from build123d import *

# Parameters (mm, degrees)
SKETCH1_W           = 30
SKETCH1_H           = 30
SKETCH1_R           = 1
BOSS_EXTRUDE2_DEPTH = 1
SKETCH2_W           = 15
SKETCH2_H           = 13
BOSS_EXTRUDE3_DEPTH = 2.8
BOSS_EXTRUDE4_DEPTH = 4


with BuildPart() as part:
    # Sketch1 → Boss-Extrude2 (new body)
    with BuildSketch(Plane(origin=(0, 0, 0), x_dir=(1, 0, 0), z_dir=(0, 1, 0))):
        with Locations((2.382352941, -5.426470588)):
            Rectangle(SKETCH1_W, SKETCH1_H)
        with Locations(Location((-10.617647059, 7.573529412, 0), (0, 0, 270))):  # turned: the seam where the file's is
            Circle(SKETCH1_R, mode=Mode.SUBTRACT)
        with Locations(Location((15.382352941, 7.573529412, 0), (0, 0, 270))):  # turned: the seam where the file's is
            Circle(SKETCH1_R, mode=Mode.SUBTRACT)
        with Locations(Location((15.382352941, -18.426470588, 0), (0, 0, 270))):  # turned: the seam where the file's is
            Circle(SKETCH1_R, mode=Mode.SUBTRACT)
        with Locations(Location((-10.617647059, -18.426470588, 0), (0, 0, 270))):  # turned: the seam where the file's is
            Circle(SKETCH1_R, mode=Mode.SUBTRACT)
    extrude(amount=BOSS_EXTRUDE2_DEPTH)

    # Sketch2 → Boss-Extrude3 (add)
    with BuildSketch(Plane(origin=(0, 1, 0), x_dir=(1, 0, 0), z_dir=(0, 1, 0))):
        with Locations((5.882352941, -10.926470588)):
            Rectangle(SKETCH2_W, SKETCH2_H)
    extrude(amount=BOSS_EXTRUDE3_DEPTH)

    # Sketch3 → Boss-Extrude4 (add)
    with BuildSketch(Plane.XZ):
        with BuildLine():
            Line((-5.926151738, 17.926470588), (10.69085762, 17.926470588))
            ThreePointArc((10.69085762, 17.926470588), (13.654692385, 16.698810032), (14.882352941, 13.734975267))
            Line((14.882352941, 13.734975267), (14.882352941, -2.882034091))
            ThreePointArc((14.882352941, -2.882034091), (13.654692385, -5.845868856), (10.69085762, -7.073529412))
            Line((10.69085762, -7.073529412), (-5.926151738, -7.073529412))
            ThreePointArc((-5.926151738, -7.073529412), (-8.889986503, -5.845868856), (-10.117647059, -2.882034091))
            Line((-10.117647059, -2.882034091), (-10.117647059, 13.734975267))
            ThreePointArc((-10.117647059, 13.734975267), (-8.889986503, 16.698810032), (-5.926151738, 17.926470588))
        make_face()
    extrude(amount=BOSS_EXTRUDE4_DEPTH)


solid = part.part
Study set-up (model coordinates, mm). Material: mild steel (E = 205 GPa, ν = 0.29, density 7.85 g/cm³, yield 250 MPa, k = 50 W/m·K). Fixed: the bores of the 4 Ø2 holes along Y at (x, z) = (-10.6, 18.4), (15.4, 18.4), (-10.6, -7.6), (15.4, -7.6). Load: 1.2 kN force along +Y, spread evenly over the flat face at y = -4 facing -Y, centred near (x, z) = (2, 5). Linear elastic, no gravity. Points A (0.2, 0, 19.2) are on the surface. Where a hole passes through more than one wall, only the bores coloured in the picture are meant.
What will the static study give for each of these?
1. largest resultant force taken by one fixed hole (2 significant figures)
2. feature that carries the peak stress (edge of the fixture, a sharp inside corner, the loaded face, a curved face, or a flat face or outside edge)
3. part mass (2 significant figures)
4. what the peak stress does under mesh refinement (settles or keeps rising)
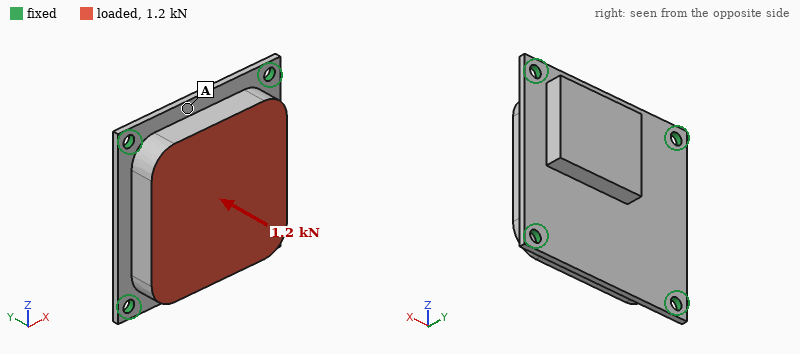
390 N
edge of the fixture
30 g
keeps rising
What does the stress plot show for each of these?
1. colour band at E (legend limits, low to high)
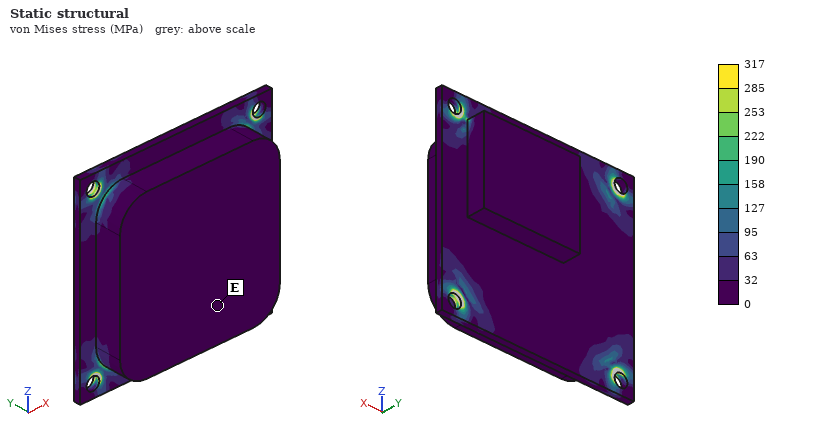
0 to 32 MPa
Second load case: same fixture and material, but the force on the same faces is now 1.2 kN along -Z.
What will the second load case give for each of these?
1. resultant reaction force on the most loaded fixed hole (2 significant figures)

350 N
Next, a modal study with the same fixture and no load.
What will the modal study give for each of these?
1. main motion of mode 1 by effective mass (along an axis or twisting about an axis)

along Y
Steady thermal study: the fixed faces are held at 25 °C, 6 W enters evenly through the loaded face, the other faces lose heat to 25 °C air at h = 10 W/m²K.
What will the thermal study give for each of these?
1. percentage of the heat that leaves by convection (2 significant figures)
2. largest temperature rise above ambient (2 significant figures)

4.2 %
17 K
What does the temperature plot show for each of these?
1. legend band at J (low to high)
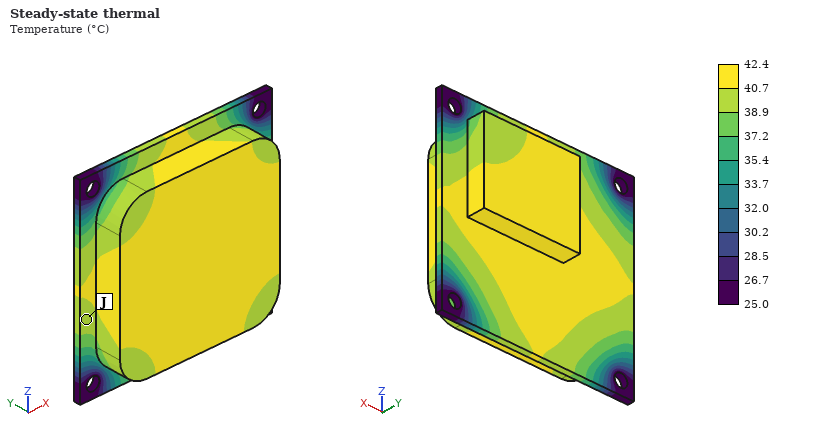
38.9 to 40.7 °C
